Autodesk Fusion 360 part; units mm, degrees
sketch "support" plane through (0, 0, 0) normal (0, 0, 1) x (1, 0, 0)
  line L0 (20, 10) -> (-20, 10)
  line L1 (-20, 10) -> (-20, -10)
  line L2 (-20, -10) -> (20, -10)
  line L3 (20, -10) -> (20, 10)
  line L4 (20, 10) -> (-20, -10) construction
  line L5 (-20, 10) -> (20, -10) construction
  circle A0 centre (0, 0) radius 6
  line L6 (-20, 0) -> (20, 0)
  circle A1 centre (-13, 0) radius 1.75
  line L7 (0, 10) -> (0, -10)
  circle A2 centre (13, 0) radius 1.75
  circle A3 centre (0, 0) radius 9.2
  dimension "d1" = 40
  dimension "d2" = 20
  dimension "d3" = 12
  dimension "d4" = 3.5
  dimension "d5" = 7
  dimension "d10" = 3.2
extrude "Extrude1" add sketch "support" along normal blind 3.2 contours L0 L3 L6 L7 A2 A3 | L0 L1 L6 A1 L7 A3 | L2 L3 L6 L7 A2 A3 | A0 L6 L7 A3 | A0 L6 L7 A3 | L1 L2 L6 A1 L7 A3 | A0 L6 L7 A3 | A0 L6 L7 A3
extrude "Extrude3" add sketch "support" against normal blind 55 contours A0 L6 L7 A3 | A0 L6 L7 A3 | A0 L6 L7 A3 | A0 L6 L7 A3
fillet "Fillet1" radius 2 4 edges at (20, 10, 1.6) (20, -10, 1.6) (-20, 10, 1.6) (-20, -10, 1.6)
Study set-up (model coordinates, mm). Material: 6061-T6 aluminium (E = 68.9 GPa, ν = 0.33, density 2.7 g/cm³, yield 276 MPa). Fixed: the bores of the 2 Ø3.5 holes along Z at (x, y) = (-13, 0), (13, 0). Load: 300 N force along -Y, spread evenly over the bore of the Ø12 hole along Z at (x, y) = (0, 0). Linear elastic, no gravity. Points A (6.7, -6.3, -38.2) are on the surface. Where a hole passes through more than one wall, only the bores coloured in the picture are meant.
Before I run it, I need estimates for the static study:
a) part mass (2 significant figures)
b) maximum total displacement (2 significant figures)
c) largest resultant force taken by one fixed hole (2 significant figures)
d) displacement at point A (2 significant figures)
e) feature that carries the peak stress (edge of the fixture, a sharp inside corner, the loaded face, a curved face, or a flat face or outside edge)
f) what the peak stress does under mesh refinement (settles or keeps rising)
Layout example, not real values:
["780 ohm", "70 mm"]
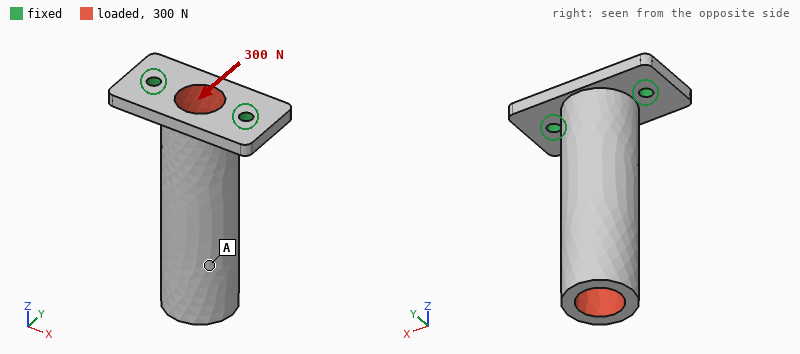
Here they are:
["28 g", "0.26 mm", "150 N", "0.18 mm", "edge of the fixture", "keeps rising"]
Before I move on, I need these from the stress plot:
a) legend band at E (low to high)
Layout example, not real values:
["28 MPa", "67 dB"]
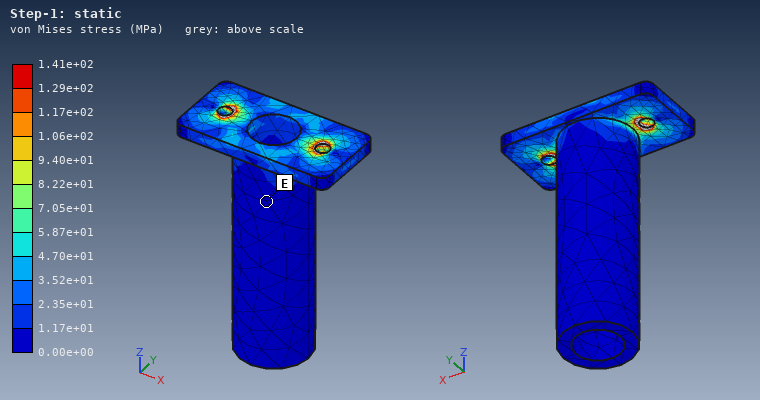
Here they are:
["0.00e+00 to 1.17e+01 MPa"]
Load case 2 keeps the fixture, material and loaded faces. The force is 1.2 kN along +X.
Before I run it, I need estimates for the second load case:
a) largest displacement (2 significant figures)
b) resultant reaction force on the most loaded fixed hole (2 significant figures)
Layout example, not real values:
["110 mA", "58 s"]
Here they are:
["0.19 mm", "1.7 kN"]
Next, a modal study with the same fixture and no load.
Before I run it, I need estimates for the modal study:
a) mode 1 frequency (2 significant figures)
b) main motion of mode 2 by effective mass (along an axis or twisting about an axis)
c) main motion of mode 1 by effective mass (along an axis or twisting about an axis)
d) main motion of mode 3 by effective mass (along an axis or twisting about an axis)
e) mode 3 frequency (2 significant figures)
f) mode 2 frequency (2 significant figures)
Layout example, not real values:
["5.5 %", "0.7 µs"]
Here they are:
["1300 Hz", "along X", "along Y", "along Z", "11 kHz", "3200 Hz"]
